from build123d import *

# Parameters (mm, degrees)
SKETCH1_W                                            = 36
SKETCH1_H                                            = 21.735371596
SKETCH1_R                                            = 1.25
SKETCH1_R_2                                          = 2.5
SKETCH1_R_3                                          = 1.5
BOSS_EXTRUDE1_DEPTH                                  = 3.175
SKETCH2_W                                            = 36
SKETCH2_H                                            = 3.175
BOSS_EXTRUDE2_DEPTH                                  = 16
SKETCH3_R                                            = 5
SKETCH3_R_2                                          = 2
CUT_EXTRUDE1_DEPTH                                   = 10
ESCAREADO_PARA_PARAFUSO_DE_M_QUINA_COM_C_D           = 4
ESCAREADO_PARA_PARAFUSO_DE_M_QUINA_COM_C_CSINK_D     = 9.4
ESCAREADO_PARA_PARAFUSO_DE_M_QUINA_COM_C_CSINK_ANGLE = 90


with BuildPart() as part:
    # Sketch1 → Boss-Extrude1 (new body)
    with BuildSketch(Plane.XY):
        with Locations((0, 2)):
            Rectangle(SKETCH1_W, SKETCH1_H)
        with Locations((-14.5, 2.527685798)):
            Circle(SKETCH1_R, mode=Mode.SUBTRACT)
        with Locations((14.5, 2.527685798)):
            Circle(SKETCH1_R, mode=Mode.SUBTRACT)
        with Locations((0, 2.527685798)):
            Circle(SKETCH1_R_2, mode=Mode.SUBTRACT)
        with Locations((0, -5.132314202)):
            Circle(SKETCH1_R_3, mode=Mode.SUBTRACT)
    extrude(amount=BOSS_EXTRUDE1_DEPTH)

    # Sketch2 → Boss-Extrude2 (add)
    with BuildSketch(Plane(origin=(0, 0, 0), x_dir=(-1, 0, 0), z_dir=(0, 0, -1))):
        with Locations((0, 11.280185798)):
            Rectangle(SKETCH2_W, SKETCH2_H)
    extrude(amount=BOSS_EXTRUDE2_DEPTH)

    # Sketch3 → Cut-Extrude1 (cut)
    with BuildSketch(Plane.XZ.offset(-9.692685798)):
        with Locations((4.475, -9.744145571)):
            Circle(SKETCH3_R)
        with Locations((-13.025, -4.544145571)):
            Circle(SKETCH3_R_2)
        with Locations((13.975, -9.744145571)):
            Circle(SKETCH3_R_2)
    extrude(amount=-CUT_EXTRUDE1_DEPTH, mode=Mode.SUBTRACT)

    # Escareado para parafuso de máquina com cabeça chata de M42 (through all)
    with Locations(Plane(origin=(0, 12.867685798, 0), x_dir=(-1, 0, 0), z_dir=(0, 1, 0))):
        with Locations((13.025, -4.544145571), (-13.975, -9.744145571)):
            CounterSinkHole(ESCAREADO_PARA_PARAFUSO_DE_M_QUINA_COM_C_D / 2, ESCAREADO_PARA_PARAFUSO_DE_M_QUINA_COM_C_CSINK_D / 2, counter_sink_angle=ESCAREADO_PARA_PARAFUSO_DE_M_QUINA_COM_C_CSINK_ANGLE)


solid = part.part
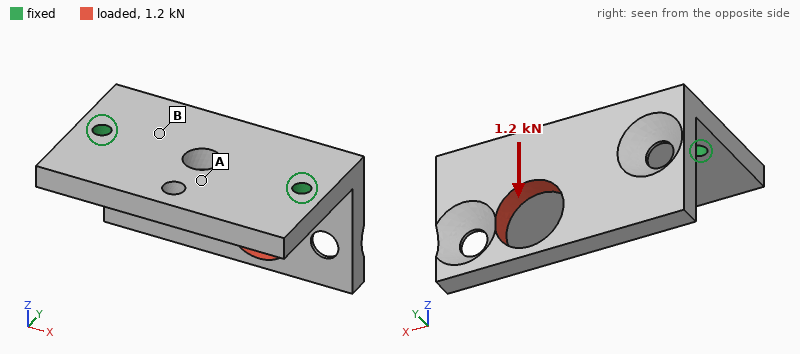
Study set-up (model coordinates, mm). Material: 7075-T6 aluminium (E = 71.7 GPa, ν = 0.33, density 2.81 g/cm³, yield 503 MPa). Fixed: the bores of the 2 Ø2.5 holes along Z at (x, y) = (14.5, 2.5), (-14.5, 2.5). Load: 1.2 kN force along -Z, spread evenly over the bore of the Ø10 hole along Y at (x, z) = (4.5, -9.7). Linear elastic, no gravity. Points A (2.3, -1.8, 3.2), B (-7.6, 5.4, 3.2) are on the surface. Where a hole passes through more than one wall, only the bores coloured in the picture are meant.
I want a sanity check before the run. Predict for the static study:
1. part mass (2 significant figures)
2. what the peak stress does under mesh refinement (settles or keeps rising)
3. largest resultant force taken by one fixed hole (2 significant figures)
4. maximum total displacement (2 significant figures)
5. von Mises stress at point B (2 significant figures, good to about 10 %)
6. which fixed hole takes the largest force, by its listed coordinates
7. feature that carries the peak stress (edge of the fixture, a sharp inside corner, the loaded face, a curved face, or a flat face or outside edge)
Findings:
10 g
keeps rising
790 N
0.21 mm
68 MPa
(14.5, 2.5)
edge of the fixture
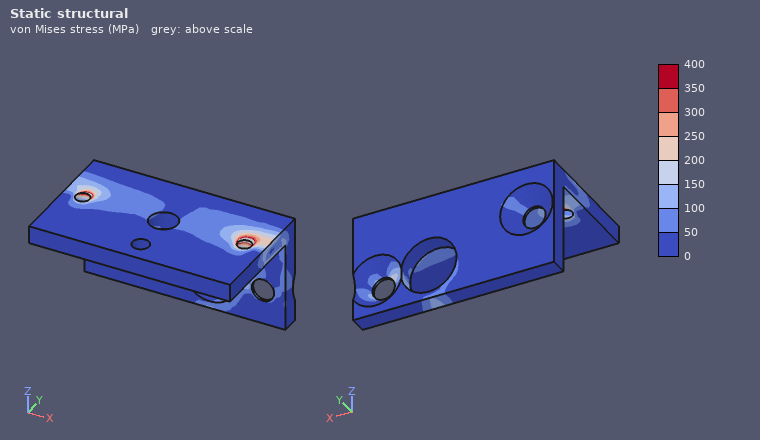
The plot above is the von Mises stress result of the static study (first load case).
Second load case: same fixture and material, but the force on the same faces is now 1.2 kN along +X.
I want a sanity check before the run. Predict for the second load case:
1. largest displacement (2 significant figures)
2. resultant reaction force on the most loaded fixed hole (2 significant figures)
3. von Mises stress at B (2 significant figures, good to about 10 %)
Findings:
86 µm
850 N
23 MPa
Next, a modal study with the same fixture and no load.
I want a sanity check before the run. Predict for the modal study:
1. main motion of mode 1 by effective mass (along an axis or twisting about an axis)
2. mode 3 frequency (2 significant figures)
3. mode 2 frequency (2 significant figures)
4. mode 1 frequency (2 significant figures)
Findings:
along Y
12 kHz
8300 Hz
4600 Hz
